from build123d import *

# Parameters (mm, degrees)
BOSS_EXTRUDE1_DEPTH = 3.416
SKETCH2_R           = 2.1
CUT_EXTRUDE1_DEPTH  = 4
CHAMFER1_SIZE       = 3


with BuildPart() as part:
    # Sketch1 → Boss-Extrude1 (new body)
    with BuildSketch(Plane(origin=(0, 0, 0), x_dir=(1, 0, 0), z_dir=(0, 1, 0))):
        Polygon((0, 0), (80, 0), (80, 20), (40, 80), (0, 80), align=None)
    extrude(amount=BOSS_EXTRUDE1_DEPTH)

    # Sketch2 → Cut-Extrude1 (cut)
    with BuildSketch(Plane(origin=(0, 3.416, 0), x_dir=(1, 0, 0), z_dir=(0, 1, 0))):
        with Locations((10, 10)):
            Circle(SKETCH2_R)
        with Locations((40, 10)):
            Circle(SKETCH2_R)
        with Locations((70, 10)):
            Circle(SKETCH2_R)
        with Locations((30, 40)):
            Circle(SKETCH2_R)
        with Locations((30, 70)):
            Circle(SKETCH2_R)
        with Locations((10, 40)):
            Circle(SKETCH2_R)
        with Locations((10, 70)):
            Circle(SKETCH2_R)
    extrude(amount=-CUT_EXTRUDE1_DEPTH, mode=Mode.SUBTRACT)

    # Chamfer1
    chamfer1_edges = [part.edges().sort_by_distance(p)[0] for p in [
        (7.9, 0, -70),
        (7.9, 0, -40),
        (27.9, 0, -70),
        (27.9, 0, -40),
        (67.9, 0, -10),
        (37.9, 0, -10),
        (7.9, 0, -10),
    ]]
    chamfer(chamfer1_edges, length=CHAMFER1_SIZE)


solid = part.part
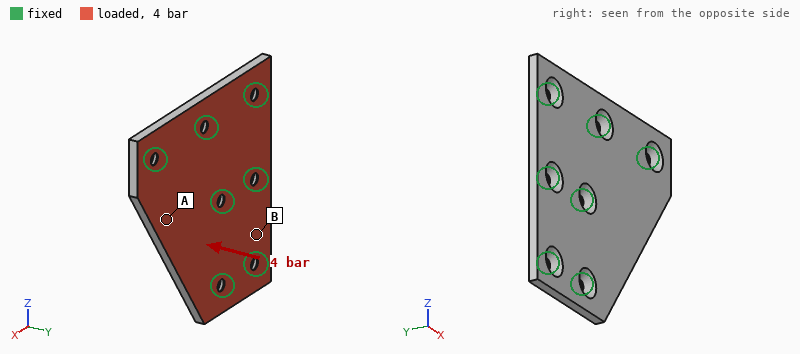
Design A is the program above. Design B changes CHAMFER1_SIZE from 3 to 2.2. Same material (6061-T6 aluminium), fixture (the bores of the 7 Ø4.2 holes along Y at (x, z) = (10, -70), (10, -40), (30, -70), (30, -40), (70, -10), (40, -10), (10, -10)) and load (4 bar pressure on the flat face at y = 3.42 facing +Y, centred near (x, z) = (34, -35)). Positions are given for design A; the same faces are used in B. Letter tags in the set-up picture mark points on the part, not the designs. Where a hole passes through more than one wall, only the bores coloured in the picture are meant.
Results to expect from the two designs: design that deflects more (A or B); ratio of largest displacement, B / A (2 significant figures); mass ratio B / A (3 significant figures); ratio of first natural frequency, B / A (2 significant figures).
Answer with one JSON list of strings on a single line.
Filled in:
["A", "0.86", "1.02", "1.1"]
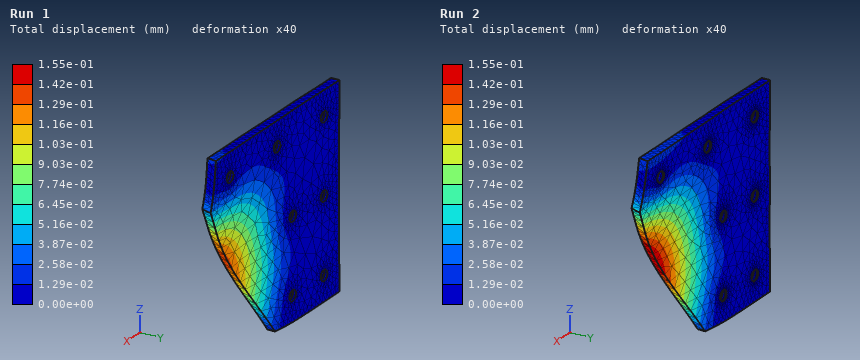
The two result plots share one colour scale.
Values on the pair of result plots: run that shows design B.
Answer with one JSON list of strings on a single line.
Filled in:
["Run 1"]
